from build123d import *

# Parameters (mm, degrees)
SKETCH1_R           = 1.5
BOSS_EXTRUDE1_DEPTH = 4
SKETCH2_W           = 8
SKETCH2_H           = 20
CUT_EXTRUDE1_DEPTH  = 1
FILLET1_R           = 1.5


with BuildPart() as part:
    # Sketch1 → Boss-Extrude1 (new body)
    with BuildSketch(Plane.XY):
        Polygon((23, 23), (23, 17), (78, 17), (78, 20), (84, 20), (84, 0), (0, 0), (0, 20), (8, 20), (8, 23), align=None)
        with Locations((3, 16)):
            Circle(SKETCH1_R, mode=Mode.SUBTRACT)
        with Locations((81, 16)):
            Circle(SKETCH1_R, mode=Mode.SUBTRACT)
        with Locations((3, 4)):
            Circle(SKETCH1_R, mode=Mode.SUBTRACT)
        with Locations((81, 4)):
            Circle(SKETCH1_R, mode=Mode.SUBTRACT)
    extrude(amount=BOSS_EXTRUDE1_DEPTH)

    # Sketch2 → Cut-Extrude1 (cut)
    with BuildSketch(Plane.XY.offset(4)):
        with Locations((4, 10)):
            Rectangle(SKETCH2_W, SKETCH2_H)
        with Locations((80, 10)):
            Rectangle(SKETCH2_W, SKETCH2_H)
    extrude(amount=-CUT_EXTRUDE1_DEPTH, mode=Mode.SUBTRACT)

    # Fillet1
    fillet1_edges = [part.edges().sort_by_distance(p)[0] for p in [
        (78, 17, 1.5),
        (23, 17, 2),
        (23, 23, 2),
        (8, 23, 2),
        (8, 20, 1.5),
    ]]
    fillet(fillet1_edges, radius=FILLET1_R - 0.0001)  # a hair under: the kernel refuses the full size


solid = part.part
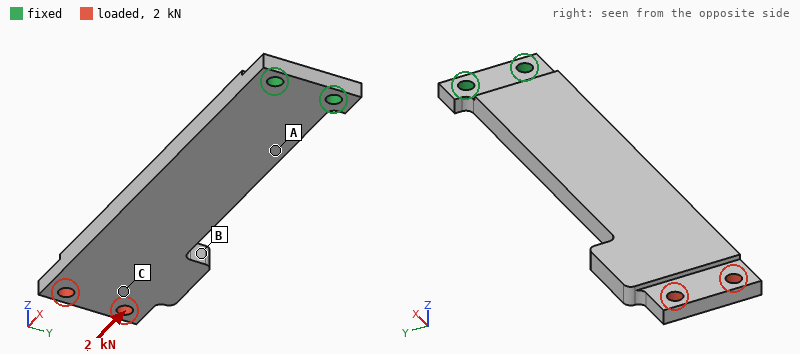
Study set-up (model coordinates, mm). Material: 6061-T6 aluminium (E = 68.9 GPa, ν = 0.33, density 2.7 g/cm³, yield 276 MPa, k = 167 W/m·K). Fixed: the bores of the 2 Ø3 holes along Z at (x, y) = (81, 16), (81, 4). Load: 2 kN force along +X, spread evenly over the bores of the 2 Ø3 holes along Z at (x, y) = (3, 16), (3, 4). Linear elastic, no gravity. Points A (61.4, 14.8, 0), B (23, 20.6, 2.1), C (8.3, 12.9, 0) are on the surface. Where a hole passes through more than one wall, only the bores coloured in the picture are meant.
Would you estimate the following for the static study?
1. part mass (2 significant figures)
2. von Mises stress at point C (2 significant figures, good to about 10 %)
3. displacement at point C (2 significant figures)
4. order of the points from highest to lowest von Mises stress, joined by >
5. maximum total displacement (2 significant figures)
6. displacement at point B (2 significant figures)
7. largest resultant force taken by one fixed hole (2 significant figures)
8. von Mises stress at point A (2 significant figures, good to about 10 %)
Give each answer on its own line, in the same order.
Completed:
16 g
35 MPa
0.37 mm
A > C > B
0.45 mm
0.22 mm
1.0 kN
63 MPa
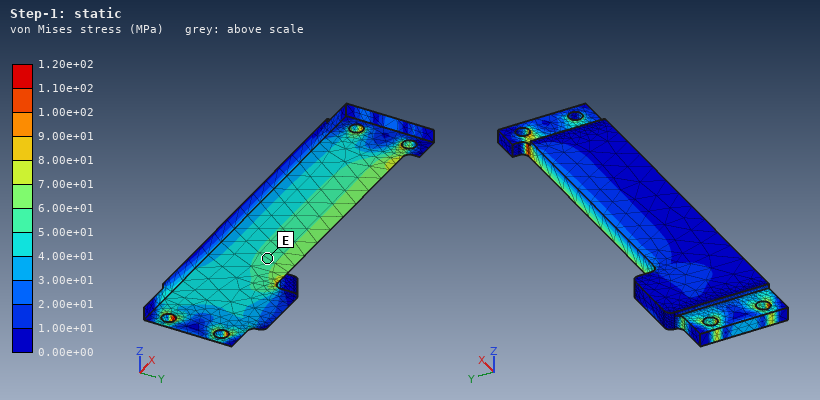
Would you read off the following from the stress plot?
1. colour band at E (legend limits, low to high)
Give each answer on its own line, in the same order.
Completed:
5.00e+01 to 6.00e+01 MPa
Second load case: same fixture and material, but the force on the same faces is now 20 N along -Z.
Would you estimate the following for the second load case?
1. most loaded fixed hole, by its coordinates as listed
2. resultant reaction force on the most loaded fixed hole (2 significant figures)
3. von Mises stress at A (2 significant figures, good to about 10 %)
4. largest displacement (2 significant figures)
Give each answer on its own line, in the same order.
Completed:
(81, 4)
13 N
26 MPa
0.66 mm
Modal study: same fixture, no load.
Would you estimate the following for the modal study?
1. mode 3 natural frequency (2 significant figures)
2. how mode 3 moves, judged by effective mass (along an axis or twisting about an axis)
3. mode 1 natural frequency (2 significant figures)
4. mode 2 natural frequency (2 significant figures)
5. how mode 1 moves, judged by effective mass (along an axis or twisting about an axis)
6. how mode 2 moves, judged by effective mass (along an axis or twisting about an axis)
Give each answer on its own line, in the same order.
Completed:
2900 Hz
along Z
420 Hz
1900 Hz
along Z
along Y
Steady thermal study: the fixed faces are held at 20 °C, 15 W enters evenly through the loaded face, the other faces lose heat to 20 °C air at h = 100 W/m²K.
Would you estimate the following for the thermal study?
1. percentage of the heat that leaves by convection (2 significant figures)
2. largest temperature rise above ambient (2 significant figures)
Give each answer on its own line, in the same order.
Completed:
64 %
57 K
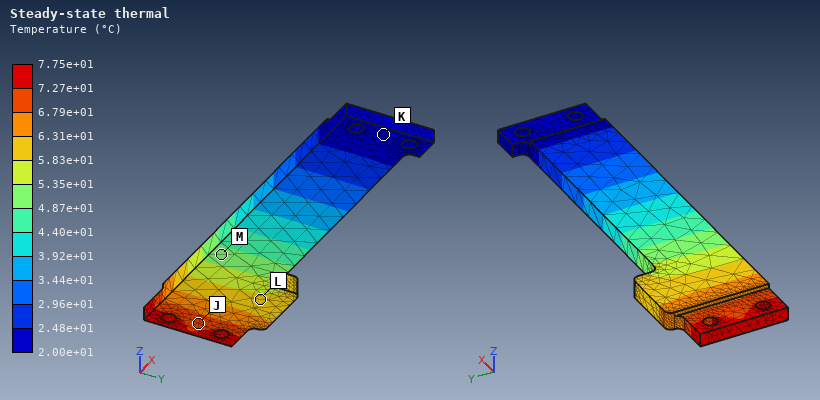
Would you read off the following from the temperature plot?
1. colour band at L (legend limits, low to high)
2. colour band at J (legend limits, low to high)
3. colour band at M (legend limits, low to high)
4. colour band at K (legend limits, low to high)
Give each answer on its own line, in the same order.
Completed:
5.83e+01 to 6.31e+01 °C
6.79e+01 to 7.27e+01 °C
4.87e+01 to 5.35e+01 °C
2.00e+01 to 2.48e+01 °C
